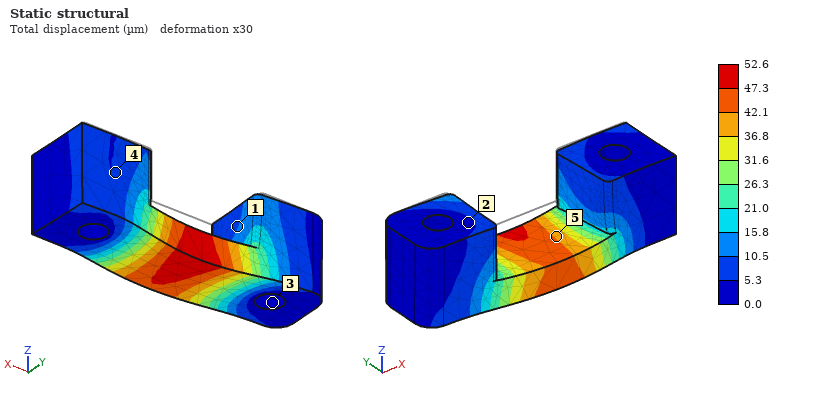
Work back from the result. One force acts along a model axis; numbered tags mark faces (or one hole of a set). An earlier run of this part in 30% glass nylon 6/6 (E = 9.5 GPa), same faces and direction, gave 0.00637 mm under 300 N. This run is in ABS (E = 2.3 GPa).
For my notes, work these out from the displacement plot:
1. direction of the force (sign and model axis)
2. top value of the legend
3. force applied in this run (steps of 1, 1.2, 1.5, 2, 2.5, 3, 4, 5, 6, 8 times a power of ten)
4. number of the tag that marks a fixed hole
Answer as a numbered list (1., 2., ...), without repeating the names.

1. -Y
2. 52.6 µm
3. 600 N
4. 3
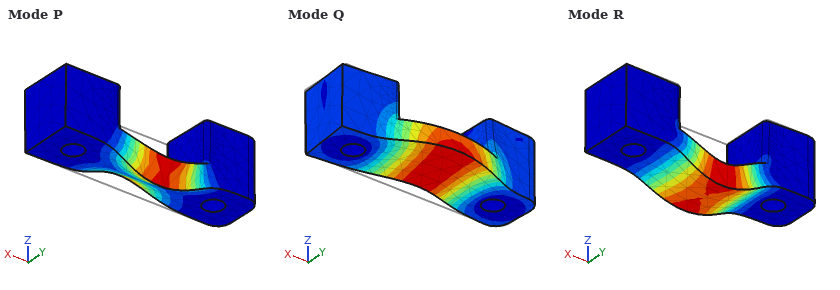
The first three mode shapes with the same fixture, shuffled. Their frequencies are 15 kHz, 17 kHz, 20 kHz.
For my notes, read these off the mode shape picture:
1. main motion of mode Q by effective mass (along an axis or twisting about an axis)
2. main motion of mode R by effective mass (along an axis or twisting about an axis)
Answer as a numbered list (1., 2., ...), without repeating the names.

1. along Y
2. along Z
